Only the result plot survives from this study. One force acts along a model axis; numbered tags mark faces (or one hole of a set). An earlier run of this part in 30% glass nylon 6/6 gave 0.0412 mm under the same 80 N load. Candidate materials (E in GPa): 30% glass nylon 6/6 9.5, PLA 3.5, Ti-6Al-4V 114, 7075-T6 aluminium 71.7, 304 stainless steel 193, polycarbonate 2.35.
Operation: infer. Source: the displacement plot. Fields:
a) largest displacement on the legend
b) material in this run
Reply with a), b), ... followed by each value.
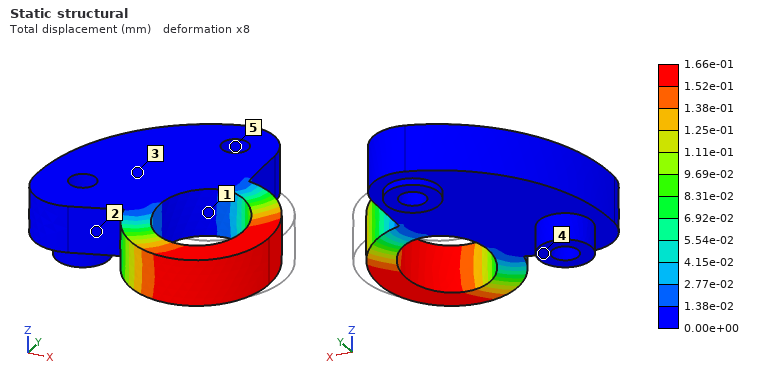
a) 1.66e-01 mm
b) polycarbonate
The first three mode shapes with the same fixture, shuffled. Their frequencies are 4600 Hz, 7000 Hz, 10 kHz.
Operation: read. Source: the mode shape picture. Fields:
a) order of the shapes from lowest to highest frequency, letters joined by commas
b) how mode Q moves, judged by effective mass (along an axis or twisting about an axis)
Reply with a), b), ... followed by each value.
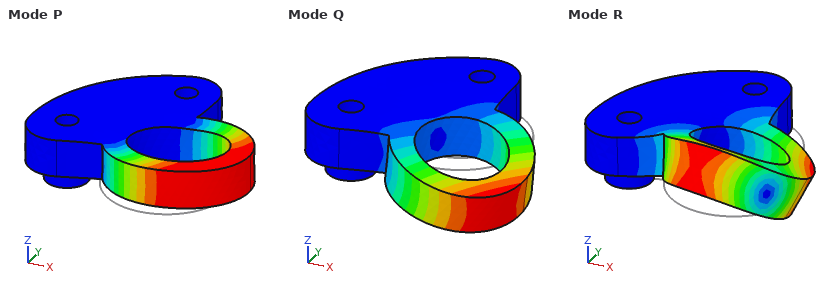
a) Q, P, R
b) along Z
